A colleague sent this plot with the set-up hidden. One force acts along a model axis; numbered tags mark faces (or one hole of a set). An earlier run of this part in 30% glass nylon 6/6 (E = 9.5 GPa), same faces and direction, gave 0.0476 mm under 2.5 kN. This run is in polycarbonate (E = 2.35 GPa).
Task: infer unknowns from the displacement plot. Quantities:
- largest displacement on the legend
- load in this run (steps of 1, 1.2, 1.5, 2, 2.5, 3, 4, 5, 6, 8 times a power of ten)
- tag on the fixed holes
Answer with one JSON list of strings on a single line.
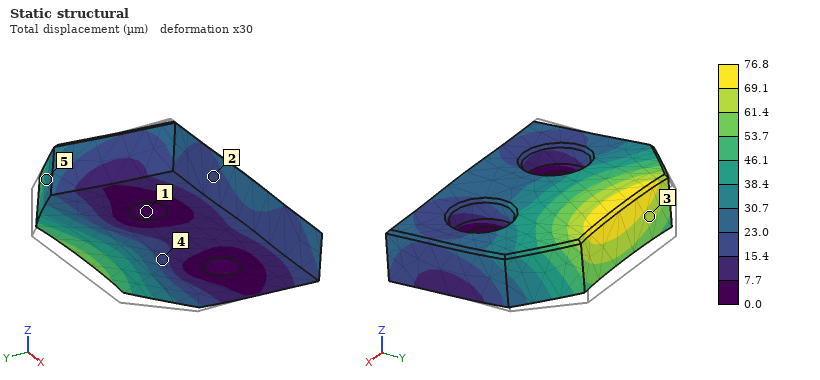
["76.8 µm", "1 kN", "1"]
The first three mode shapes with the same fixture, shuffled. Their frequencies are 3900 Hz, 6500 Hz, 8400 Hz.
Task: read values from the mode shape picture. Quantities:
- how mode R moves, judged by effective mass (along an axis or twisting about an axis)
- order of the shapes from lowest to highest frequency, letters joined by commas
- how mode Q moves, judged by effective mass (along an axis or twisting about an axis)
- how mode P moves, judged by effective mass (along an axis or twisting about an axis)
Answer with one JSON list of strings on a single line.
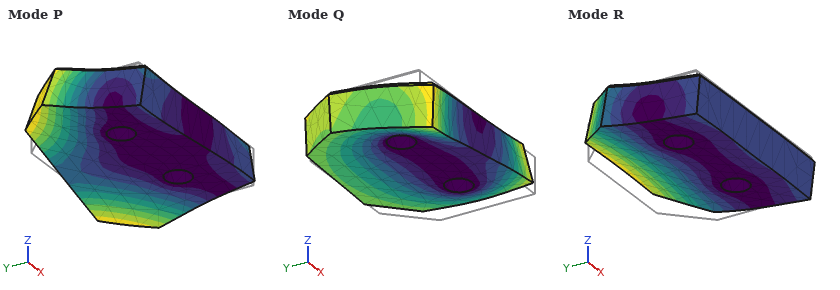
["along Z", "R, P, Q", "along X", "twisting about Y"]
